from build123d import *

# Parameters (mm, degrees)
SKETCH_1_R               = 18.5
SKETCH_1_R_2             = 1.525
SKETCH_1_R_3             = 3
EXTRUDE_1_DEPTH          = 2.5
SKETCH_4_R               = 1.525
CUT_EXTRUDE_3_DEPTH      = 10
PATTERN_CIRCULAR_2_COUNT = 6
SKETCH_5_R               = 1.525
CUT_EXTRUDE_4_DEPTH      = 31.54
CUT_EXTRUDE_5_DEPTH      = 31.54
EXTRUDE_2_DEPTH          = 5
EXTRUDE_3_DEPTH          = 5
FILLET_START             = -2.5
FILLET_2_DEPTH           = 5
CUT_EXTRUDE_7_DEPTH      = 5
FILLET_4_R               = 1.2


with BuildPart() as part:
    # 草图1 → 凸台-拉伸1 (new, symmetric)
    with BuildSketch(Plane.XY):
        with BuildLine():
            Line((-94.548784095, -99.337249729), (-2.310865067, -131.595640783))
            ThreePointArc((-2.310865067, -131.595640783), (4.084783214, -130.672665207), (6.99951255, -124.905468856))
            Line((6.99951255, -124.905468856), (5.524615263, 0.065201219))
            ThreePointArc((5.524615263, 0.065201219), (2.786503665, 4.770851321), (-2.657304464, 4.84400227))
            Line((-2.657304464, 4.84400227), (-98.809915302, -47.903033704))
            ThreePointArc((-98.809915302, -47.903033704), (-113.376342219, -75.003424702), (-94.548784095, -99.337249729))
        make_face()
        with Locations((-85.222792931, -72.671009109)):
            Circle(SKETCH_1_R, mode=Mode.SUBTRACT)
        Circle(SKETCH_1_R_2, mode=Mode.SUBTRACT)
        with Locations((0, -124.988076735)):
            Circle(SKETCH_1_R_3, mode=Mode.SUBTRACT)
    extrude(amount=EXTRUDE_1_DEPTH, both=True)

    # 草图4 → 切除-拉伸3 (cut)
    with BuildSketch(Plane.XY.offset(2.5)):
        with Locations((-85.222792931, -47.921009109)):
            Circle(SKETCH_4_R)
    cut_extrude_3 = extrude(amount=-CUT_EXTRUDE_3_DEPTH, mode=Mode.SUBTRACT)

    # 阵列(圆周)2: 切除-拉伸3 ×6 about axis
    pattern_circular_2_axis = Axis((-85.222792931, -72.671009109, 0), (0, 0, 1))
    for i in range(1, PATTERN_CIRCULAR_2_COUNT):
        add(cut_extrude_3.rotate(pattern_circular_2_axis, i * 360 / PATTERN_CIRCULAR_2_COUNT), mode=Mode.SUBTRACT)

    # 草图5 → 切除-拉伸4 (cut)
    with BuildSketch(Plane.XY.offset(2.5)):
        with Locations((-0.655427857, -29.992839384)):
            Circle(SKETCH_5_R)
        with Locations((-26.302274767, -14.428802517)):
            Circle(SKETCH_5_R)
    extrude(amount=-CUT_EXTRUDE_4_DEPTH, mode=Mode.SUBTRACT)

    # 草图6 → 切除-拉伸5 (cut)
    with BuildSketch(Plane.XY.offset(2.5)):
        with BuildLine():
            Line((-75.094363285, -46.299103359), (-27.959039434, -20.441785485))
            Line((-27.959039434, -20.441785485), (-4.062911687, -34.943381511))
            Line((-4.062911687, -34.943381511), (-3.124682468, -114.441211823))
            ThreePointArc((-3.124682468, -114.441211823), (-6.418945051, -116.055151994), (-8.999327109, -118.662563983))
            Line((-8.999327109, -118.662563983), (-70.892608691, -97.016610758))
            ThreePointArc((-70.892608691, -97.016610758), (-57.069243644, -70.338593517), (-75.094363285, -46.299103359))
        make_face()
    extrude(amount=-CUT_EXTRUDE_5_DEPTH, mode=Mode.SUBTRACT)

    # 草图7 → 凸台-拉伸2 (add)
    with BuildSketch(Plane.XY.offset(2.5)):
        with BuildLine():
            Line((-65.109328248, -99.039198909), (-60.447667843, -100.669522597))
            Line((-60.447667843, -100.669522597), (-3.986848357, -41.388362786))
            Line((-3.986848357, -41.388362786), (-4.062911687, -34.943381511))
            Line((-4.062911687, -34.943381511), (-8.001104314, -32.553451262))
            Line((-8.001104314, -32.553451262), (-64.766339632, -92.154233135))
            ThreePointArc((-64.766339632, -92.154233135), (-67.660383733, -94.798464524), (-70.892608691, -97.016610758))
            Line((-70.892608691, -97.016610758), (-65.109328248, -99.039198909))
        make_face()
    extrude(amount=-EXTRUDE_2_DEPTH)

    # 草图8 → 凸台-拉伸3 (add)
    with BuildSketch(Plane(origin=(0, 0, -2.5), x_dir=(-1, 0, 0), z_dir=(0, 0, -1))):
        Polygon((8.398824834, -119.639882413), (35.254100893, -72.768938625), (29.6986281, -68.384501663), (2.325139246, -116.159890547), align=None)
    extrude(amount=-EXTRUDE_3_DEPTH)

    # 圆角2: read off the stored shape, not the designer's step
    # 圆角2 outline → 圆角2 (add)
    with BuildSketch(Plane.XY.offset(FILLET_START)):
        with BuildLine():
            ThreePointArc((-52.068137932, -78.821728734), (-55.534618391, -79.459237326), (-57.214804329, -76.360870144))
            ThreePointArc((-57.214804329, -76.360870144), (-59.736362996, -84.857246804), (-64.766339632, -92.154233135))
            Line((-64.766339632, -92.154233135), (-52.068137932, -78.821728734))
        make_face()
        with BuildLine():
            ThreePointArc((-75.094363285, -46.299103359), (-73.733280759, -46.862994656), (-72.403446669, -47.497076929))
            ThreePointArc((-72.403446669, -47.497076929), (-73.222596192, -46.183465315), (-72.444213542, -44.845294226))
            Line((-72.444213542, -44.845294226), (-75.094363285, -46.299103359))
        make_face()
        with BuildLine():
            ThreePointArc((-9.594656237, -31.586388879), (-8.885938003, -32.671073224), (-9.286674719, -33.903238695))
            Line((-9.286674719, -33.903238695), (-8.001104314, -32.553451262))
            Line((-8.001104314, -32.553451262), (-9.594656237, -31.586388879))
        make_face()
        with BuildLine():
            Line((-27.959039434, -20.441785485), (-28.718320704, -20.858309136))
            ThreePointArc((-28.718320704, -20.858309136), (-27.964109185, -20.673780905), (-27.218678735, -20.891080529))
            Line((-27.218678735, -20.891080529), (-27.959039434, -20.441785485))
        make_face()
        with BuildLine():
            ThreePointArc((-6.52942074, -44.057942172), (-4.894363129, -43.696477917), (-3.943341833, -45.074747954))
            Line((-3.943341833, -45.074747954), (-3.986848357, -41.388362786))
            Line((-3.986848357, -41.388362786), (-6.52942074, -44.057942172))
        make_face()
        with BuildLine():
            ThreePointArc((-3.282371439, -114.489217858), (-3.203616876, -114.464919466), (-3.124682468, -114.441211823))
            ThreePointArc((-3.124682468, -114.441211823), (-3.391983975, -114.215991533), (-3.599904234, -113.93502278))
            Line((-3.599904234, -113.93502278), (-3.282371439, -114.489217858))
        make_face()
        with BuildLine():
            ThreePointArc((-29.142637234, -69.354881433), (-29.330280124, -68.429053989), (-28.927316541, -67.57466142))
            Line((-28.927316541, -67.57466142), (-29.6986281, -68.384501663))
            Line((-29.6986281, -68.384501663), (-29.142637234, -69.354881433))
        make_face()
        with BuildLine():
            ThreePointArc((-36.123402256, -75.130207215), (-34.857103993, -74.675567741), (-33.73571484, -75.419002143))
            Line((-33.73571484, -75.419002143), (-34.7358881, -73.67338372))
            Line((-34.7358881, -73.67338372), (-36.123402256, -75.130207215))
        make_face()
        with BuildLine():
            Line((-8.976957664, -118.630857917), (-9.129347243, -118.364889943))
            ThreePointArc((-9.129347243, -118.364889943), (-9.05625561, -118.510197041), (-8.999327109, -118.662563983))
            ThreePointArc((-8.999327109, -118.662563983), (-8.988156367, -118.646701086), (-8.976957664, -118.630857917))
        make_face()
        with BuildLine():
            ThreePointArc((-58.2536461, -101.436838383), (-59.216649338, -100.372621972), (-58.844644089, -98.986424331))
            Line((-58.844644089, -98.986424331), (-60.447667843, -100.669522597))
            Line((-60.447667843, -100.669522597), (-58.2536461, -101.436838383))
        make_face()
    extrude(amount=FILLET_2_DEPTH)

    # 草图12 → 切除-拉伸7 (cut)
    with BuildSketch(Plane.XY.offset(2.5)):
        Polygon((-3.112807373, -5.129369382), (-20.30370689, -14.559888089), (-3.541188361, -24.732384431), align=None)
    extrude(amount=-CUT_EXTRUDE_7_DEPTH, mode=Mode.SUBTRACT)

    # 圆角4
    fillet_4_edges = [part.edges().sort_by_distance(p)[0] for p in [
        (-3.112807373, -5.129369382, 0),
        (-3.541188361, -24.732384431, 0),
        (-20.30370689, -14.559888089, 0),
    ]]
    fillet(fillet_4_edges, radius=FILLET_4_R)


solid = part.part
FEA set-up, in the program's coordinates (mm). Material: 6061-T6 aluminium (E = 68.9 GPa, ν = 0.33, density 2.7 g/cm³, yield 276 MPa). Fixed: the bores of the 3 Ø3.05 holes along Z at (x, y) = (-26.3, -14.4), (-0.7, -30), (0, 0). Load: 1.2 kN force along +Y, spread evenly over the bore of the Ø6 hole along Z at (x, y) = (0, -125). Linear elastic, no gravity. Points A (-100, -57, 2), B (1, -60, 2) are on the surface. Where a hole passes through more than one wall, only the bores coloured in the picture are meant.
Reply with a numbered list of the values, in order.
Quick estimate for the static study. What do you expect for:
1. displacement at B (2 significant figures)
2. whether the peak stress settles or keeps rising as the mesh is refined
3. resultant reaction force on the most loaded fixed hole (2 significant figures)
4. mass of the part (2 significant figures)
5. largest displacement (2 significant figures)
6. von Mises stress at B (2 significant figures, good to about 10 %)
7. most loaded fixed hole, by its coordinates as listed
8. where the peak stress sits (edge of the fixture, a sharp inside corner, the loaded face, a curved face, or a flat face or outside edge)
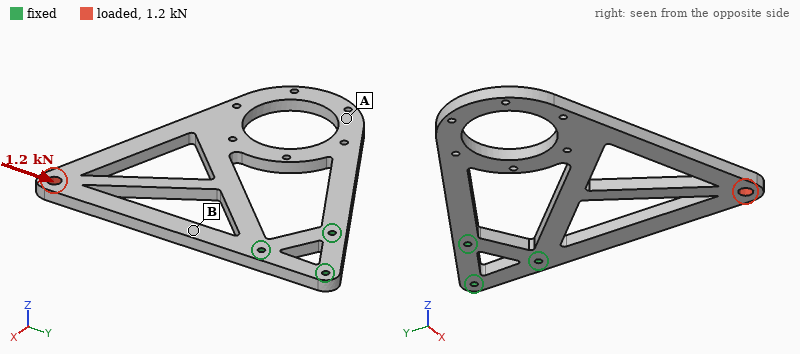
1. 11 µm
2. keeps rising
3. 1.1 kN
4. 78 g
5. 36 µm
6. 21 MPa
7. (-0.7, -30)
8. edge of the fixture
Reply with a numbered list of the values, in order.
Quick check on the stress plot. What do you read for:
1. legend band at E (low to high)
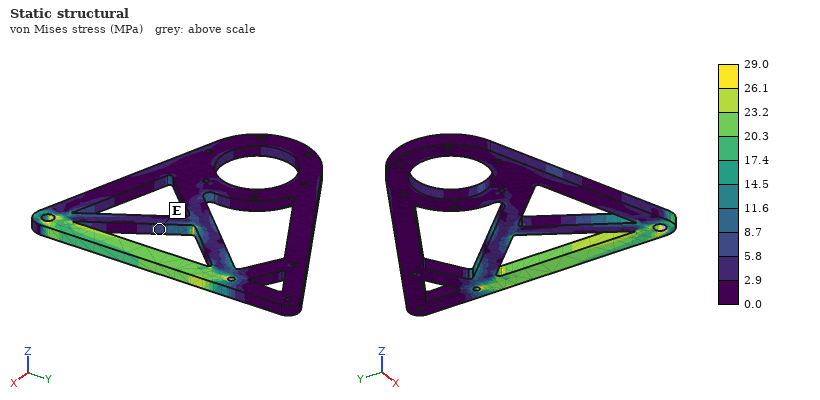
1. 5.8 to 8.7 MPa
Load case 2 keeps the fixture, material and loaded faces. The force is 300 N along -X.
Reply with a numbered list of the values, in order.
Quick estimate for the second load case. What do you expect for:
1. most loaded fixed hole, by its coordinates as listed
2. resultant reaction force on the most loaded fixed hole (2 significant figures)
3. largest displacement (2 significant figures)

1. (-0.7, -30)
2. 760 N
3. 0.37 mm
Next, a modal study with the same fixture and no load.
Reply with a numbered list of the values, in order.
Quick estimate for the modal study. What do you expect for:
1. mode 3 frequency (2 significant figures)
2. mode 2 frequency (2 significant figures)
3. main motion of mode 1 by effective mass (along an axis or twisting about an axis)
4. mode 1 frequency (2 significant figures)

1. 750 Hz
2. 430 Hz
3. along Z
4. 230 Hz
